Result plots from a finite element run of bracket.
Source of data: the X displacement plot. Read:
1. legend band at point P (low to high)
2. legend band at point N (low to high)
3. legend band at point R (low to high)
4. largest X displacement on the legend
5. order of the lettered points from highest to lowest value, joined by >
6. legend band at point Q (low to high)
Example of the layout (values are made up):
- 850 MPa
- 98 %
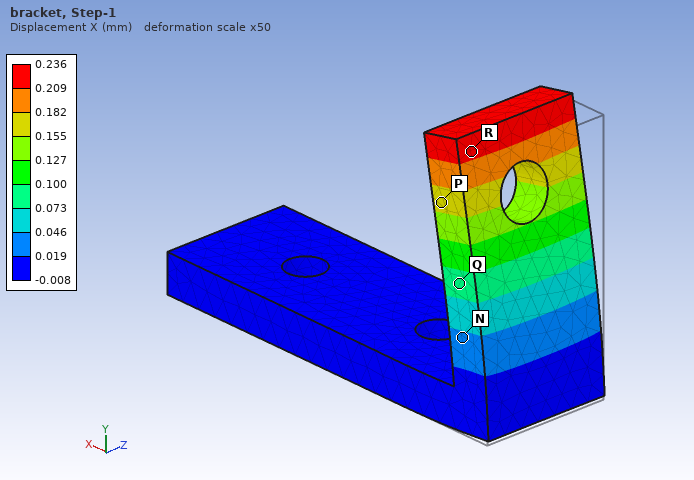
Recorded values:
- 0.155 to 0.182 mm
- 0.019 to 0.046 mm
- 0.209 to 0.236 mm
- 0.236 mm
- R > P > Q > N
- 0.073 to 0.100 mm
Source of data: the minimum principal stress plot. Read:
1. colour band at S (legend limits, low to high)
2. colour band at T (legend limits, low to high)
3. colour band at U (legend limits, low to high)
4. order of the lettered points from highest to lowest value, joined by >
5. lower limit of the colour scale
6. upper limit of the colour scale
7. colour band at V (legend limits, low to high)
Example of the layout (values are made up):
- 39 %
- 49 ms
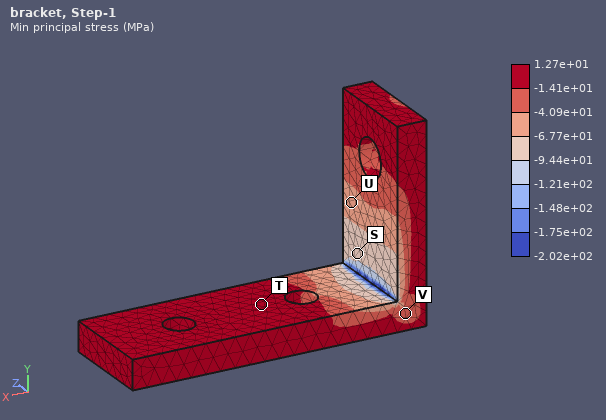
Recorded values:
- -9.44e+01 to -6.77e+01 MPa
- -1.41e+01 to 1.27e+01 MPa
- -6.77e+01 to -4.09e+01 MPa
- T > V > U > S
- -2.02e+02 MPa
- 1.27e+01 MPa
- -4.09e+01 to -1.41e+01 MPa
